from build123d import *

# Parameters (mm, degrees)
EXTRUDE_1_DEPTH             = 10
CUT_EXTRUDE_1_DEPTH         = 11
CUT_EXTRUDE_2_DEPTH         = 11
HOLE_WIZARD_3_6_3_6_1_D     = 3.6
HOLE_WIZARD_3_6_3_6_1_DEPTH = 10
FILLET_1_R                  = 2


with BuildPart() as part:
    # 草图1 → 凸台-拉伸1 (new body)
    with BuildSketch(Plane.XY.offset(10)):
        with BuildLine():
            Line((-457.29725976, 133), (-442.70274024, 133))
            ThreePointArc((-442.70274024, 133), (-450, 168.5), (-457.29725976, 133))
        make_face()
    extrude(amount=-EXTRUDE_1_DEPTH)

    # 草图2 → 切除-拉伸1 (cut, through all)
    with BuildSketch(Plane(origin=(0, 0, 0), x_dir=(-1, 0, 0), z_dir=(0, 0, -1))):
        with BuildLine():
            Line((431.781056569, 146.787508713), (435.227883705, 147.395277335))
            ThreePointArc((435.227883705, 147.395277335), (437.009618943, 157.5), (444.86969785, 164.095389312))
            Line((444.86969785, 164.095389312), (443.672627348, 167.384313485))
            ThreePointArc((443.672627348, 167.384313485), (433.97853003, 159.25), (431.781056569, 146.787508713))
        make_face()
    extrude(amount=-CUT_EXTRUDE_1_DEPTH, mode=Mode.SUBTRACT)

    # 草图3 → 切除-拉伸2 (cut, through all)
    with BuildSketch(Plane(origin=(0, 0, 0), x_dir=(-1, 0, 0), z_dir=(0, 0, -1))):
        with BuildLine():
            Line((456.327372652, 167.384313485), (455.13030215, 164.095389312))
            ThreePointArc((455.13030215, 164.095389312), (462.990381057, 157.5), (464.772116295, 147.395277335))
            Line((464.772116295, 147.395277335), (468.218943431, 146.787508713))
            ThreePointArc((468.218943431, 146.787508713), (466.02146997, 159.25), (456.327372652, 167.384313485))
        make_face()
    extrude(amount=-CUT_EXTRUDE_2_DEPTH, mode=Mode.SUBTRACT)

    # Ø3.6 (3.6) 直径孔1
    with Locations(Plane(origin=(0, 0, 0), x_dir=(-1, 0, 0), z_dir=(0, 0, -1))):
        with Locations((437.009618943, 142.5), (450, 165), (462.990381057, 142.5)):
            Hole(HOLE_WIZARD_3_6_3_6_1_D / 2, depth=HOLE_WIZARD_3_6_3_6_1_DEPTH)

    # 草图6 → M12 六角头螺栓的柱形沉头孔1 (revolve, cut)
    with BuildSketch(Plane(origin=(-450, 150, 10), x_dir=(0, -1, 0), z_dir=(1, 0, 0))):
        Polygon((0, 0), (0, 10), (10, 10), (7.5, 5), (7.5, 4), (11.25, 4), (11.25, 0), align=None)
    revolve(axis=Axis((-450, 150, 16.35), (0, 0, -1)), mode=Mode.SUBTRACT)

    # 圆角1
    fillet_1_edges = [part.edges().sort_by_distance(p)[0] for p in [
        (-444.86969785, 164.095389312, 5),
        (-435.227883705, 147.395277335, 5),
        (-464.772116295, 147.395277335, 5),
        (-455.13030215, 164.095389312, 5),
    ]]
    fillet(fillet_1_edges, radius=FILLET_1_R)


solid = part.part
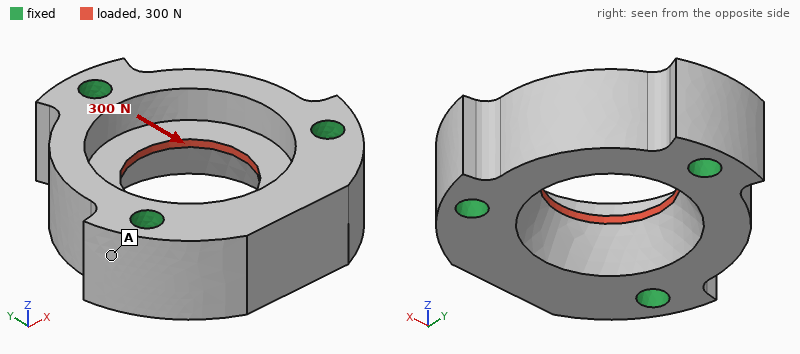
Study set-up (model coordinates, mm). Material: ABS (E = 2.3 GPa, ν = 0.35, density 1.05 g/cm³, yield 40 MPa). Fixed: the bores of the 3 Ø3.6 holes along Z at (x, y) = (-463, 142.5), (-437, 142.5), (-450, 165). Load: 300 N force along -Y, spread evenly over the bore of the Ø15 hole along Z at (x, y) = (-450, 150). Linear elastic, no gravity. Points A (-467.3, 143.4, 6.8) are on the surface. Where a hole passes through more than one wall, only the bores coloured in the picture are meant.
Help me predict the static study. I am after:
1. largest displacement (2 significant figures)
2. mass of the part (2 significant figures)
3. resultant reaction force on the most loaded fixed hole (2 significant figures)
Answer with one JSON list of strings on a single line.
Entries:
["21 µm", "6.0 g", "110 N"]
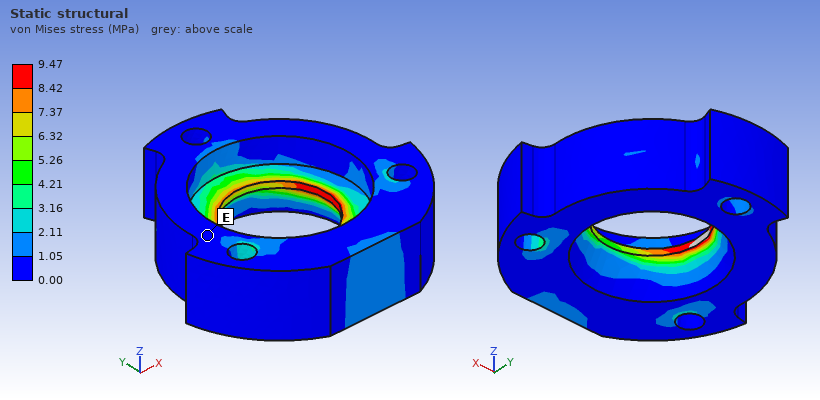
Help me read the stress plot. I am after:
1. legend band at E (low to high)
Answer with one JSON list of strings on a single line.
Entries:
["0.00 to 1.05 MPa"]
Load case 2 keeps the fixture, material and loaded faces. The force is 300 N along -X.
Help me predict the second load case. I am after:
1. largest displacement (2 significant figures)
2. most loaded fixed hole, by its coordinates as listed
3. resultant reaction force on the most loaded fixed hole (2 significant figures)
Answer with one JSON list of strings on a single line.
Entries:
["23 µm", "(-450, 165)", "120 N"]
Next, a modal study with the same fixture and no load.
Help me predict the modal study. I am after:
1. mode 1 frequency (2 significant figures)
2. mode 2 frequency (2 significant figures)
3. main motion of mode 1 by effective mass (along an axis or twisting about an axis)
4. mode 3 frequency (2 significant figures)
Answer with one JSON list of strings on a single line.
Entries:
["11 kHz", "12 kHz", "along Z", "13 kHz"]
